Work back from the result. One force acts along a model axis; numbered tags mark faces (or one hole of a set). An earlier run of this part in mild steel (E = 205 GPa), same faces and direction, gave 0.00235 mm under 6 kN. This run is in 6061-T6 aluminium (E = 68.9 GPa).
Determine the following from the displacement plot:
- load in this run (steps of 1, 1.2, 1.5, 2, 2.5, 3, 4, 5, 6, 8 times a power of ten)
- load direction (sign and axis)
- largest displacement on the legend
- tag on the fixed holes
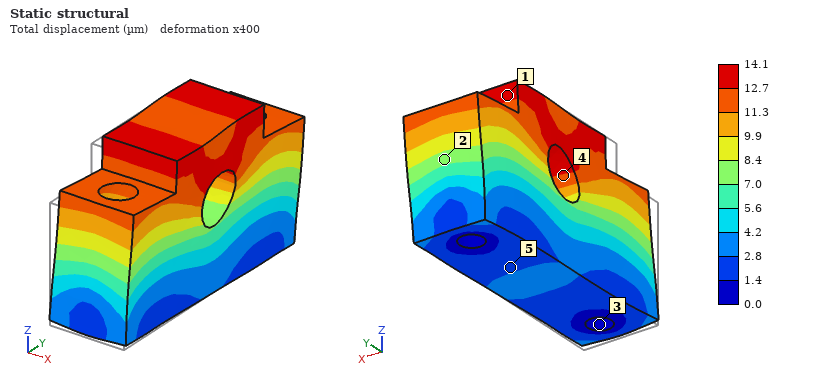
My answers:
12 kN
+Y
14.1 µm
3
